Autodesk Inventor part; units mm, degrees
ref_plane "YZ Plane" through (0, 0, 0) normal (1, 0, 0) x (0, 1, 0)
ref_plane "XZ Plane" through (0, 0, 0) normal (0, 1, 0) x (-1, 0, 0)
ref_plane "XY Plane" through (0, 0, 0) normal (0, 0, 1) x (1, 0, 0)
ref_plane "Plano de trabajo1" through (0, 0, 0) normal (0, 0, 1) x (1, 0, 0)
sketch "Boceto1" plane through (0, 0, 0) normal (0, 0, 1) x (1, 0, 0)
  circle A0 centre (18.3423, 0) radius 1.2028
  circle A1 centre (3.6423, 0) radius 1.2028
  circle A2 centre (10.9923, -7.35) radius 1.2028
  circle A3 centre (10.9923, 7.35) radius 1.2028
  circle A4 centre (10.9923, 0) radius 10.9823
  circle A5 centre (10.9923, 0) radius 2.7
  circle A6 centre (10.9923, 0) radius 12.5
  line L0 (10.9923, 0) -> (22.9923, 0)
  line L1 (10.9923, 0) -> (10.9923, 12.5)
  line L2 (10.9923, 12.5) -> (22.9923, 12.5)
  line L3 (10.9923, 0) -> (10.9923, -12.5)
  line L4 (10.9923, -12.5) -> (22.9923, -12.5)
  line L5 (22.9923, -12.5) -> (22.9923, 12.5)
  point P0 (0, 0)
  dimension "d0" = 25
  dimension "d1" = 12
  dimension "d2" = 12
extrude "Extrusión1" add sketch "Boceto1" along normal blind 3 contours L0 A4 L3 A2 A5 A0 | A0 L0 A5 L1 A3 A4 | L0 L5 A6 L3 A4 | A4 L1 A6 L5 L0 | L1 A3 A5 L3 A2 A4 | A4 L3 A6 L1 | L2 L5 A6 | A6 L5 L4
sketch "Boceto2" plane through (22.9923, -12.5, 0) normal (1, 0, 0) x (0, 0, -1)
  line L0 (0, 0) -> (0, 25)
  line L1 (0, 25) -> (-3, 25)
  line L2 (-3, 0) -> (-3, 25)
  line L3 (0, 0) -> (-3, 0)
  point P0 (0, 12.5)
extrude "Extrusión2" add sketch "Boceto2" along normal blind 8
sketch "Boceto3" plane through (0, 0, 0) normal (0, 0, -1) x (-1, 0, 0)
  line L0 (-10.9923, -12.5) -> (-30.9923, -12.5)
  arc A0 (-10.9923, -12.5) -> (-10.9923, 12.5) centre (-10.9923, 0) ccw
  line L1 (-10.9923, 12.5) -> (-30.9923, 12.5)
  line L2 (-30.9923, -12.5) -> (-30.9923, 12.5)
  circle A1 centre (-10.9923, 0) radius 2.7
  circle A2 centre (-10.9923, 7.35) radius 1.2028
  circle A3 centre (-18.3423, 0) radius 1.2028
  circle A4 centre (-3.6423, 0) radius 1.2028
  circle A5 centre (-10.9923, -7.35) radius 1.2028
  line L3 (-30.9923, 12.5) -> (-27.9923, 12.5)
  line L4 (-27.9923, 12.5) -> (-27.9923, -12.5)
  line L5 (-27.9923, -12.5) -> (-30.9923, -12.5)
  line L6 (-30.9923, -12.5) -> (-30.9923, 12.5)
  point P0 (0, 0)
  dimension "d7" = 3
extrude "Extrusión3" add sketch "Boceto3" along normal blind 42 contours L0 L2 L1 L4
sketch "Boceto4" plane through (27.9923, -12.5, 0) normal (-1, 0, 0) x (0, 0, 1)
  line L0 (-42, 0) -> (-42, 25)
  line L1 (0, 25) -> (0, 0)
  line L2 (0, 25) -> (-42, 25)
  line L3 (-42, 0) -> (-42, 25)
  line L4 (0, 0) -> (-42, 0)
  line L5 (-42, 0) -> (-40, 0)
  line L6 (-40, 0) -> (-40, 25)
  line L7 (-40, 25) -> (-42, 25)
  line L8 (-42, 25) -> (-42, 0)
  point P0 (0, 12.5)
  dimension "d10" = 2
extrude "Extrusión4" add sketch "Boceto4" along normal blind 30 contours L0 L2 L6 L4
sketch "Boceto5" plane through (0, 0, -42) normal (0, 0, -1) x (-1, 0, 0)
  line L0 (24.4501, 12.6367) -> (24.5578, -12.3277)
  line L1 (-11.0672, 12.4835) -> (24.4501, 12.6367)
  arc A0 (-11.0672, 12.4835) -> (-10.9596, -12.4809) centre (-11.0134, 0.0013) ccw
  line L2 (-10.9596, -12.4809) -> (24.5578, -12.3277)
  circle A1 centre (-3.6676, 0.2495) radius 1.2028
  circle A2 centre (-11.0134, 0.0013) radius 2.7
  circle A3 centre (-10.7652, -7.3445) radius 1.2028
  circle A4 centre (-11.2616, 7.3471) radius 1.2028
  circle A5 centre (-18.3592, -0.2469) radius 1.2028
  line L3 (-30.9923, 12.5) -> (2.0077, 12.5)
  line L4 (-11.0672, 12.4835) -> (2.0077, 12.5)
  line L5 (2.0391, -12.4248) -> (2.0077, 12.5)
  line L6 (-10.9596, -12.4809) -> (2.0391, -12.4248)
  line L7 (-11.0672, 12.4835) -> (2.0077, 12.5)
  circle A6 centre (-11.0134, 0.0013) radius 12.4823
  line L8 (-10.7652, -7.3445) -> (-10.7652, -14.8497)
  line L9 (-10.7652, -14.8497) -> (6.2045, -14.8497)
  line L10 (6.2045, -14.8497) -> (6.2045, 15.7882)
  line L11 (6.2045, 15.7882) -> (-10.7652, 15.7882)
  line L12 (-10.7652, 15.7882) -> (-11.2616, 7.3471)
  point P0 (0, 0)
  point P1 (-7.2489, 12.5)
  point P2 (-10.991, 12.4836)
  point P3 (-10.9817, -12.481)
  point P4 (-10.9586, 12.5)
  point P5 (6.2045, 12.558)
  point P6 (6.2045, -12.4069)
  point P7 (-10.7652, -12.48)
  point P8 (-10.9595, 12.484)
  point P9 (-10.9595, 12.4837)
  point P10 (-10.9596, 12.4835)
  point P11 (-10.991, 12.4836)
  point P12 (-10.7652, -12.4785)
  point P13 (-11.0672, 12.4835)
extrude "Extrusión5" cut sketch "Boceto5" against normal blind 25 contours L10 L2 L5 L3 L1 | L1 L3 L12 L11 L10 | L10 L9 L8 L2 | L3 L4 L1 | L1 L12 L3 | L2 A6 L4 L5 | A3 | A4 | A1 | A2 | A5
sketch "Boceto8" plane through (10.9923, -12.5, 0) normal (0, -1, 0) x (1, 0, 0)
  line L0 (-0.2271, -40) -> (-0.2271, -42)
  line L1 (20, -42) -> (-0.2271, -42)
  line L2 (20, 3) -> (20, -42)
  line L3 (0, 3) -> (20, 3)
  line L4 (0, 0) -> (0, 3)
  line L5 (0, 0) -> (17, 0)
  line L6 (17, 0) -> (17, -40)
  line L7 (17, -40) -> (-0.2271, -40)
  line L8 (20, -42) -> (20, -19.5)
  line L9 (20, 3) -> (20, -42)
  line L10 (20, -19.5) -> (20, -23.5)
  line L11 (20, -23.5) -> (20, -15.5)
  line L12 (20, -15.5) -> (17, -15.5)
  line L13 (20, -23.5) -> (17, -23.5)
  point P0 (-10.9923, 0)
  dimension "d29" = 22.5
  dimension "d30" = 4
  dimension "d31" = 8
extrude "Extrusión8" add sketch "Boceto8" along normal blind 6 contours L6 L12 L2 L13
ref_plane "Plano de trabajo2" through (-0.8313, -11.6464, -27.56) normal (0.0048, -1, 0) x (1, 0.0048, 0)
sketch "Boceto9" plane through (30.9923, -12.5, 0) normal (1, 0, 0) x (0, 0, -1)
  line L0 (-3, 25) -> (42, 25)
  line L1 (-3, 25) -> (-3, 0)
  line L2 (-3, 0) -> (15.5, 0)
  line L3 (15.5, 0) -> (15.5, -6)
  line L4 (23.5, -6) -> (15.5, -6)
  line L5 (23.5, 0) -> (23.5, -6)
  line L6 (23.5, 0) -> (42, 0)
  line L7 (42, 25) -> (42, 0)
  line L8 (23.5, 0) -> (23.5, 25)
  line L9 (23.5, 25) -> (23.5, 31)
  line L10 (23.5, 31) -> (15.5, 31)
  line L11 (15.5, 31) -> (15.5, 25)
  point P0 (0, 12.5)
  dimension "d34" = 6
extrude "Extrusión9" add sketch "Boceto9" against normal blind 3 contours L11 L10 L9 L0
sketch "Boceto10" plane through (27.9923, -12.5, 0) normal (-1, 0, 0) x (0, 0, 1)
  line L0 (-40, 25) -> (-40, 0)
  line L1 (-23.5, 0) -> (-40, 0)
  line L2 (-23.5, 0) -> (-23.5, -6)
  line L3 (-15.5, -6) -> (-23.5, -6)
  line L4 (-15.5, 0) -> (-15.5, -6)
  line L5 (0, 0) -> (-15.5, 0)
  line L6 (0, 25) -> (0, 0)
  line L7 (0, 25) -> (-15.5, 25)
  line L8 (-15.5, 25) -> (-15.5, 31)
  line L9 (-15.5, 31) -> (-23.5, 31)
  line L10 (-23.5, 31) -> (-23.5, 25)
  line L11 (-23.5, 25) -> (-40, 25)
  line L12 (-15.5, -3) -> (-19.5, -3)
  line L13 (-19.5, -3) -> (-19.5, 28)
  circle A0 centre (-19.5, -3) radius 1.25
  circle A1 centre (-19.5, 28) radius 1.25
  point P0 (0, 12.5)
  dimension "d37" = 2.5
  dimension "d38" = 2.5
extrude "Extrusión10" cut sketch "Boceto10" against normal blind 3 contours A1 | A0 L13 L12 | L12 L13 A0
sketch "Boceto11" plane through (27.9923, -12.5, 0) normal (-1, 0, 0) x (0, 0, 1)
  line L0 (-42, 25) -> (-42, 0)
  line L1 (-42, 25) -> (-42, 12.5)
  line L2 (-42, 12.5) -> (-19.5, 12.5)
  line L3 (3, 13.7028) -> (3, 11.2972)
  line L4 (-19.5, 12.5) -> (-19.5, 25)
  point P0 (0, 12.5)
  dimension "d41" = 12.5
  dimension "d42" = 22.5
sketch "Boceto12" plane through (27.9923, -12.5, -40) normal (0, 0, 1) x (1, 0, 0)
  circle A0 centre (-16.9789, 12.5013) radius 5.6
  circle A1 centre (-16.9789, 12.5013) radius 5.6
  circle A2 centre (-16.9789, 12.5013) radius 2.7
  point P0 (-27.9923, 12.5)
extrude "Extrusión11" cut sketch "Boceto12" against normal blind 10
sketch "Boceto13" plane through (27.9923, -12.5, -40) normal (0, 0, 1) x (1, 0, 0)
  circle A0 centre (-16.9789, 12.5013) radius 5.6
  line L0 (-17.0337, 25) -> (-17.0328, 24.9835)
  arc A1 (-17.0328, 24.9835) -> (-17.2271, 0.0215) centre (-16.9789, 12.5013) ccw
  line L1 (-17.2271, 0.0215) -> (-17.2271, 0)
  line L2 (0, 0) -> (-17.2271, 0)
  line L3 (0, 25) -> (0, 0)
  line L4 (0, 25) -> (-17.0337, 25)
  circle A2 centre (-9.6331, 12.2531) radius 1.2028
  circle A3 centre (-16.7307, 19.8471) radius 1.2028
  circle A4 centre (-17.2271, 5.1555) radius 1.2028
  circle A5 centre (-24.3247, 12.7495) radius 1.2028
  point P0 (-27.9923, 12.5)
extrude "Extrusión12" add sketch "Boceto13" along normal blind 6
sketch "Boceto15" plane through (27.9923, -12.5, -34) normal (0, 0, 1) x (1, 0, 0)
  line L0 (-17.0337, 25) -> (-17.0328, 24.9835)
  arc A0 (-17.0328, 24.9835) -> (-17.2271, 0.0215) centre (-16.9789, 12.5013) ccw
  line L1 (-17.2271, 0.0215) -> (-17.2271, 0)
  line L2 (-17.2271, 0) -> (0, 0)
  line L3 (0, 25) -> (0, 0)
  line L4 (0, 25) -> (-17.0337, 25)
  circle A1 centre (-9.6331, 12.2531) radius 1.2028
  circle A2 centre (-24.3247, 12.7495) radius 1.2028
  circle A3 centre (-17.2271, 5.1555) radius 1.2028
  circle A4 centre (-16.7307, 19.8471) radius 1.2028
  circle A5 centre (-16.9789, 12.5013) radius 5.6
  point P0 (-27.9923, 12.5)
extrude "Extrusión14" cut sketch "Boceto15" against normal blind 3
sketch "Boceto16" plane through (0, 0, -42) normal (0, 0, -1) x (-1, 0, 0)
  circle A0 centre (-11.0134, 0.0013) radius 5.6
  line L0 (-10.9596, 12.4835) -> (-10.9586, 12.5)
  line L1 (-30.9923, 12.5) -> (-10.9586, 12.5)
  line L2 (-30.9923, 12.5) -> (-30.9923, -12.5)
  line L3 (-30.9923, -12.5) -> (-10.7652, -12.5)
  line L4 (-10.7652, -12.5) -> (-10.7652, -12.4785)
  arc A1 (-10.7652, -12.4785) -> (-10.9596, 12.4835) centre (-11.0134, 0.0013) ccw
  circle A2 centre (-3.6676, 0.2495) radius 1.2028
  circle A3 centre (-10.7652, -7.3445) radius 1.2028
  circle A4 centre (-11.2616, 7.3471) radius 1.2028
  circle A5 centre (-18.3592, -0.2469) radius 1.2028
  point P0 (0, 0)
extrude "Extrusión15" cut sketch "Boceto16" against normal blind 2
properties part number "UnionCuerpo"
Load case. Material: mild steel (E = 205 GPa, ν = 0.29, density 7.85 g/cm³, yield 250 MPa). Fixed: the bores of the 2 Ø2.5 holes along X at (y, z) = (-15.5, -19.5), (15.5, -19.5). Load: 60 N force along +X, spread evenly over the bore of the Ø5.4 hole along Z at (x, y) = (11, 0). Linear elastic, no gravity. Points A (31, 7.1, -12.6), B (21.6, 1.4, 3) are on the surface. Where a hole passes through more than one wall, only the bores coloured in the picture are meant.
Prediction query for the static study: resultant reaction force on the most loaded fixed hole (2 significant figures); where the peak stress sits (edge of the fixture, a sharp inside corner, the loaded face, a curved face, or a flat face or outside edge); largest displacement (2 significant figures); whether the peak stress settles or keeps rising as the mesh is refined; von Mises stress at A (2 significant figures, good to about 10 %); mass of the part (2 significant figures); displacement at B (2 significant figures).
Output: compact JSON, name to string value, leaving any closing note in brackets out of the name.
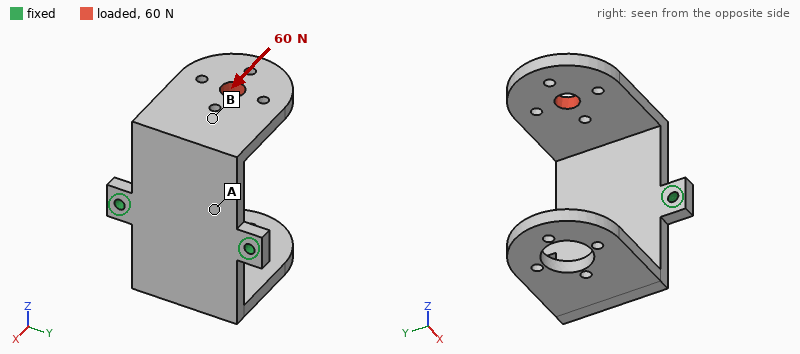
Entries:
{"resultant reaction force on the most loaded fixed hole": "30 N", "where the peak stress sits": "edge of the fixture", "largest displacement": "59 µm", "whether the peak stress settles or keeps rising as the mesh is refined": "keeps rising", "von Mises stress at A": "24 MPa", "mass of the part": "55 g", "displacement at B": "32 µm"}
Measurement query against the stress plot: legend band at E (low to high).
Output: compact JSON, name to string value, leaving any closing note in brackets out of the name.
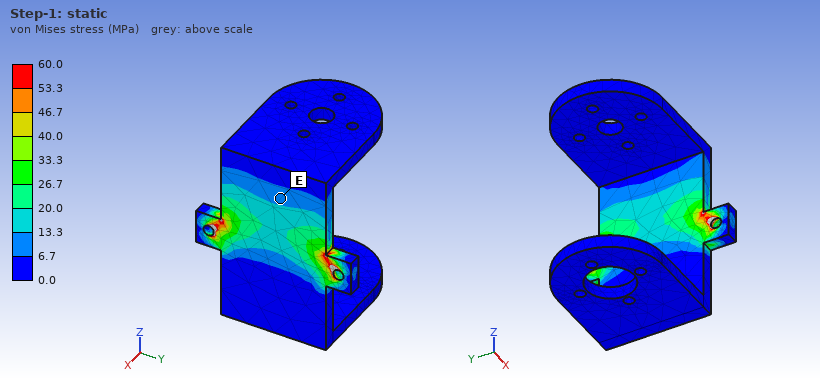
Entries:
{"legend band at E": "6.7 to 13.3 MPa"}
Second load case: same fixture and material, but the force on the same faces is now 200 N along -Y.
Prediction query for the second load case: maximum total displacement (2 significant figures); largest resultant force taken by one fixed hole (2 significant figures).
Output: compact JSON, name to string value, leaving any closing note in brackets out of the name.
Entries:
{"maximum total displacement": "90 µm", "largest resultant force taken by one fixed hole": "230 N"}
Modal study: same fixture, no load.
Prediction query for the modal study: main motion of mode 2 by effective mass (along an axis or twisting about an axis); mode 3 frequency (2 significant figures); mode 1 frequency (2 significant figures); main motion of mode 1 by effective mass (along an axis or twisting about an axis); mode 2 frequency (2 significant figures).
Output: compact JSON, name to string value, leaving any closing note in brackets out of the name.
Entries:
{"main motion of mode 2 by effective mass": "along X", "mode 3 frequency": "2500 Hz", "mode 1 frequency": "1100 Hz", "main motion of mode 1 by effective mass": "along Z", "mode 2 frequency": "1500 Hz"}
